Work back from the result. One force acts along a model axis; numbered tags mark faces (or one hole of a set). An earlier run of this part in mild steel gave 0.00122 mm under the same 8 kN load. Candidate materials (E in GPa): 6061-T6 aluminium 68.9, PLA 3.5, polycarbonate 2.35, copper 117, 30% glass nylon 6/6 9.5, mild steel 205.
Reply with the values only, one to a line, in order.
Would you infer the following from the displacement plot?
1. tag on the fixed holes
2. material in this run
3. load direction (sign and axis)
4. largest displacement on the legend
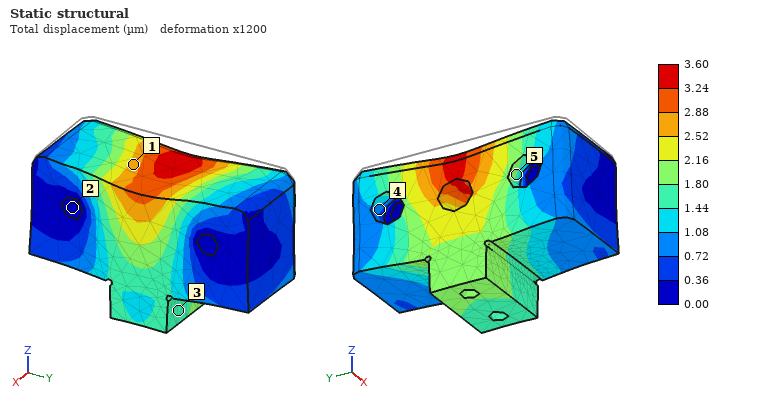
2
6061-T6 aluminium
-Z
3.60 µm
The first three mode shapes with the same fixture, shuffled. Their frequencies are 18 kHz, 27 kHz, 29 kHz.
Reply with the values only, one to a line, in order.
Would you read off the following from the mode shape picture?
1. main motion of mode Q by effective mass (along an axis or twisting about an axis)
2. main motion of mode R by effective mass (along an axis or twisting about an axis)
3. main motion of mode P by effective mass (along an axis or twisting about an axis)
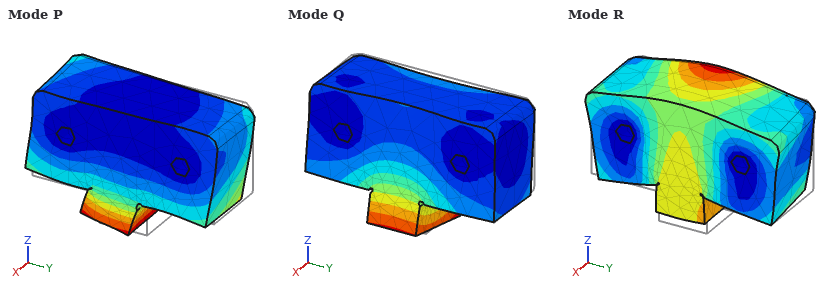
along X
along Z
along Y
